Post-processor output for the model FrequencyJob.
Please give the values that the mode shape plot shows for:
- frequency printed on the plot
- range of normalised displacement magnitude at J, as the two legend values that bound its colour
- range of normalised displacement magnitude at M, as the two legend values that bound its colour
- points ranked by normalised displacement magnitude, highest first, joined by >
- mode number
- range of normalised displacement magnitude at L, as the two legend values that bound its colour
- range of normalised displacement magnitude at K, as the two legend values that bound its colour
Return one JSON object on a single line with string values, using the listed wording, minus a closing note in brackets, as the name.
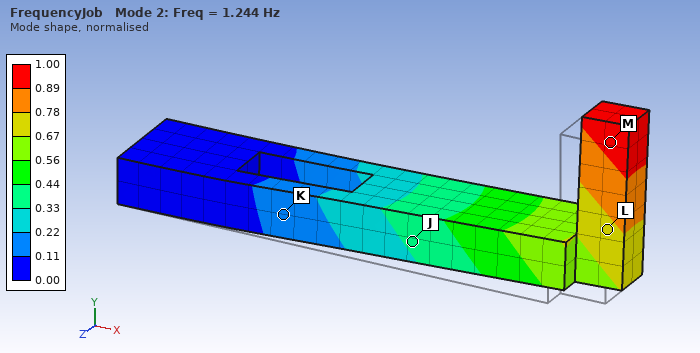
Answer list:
{"frequency printed on the plot": "1.244 Hz", "range of normalised displacement magnitude at J, as the two legend values that bound its colour": "0.33 to 0.44", "range of normalised displacement magnitude at M, as the two legend values that bound its colour": "0.89 to 1.00", "points ranked by normalised displacement magnitude, highest first, joined by >": "M > L > J > K", "mode number": "2", "range of normalised displacement magnitude at L, as the two legend values that bound its colour": "0.67 to 0.78", "range of normalised displacement magnitude at K, as the two legend values that bound its colour": "0.11 to 0.22"}
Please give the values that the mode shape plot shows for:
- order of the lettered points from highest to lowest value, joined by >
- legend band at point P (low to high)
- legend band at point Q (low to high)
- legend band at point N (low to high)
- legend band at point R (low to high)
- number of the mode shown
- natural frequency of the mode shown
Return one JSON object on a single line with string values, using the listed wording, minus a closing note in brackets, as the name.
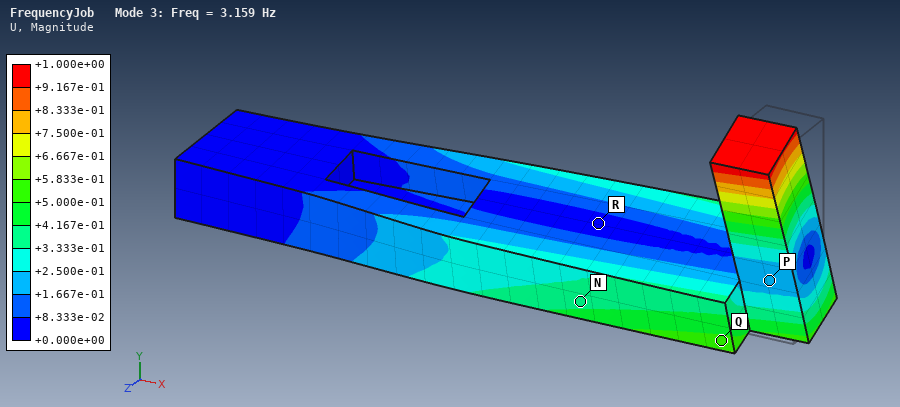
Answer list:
{"order of the lettered points from highest to lowest value, joined by >": "Q > N > P > R", "legend band at point P": "+1.667e-01 to +2.500e-01", "legend band at point Q": "+5.000e-01 to +5.833e-01", "legend band at point N": "+3.333e-01 to +4.167e-01", "legend band at point R": "+0.000e+00 to +8.333e-02", "number of the mode shown": "3", "natural frequency of the mode shown": "3.159 Hz"}
